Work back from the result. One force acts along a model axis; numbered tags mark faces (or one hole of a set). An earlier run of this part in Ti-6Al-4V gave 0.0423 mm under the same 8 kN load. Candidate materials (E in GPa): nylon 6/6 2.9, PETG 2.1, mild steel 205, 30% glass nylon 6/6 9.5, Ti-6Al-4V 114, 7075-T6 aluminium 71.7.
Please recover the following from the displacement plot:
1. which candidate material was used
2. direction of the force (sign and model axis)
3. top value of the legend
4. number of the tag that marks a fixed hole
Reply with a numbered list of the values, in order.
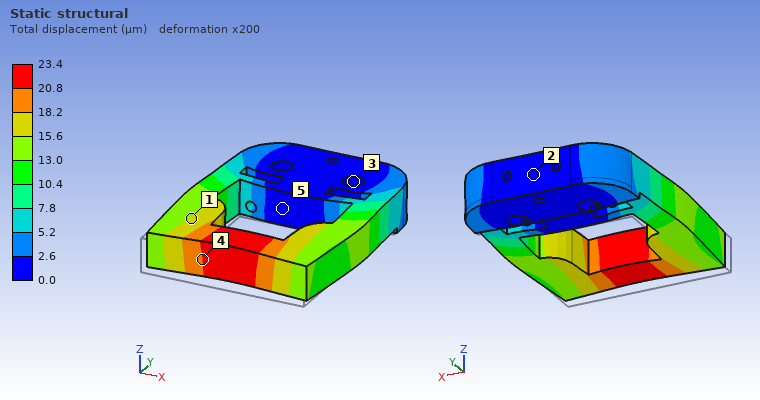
1. mild steel
2. +Y
3. 23.4 µm
4. 3
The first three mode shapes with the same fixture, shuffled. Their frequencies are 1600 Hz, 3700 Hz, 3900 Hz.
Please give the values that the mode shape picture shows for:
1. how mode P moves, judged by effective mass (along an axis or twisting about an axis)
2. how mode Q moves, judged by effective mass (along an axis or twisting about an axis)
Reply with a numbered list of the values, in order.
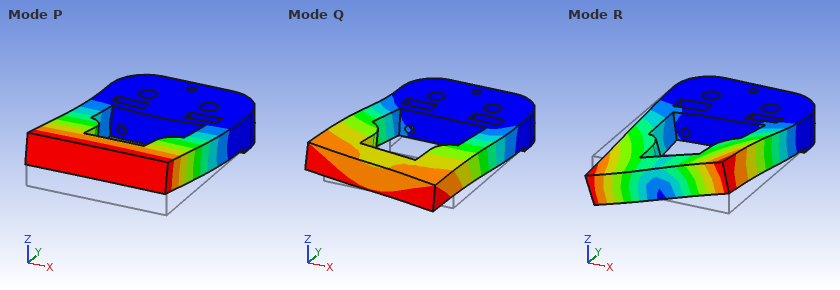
1. along Z
2. along X
